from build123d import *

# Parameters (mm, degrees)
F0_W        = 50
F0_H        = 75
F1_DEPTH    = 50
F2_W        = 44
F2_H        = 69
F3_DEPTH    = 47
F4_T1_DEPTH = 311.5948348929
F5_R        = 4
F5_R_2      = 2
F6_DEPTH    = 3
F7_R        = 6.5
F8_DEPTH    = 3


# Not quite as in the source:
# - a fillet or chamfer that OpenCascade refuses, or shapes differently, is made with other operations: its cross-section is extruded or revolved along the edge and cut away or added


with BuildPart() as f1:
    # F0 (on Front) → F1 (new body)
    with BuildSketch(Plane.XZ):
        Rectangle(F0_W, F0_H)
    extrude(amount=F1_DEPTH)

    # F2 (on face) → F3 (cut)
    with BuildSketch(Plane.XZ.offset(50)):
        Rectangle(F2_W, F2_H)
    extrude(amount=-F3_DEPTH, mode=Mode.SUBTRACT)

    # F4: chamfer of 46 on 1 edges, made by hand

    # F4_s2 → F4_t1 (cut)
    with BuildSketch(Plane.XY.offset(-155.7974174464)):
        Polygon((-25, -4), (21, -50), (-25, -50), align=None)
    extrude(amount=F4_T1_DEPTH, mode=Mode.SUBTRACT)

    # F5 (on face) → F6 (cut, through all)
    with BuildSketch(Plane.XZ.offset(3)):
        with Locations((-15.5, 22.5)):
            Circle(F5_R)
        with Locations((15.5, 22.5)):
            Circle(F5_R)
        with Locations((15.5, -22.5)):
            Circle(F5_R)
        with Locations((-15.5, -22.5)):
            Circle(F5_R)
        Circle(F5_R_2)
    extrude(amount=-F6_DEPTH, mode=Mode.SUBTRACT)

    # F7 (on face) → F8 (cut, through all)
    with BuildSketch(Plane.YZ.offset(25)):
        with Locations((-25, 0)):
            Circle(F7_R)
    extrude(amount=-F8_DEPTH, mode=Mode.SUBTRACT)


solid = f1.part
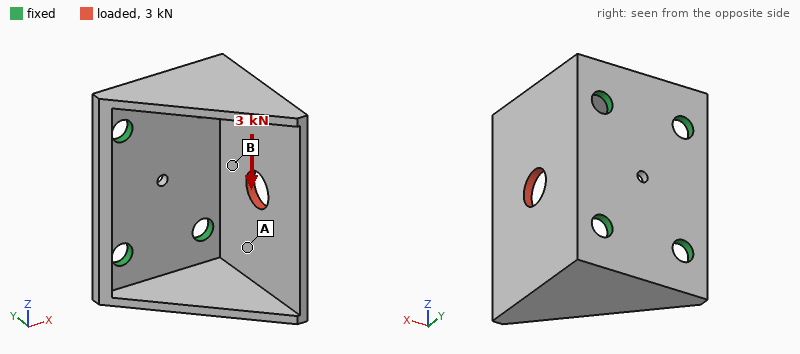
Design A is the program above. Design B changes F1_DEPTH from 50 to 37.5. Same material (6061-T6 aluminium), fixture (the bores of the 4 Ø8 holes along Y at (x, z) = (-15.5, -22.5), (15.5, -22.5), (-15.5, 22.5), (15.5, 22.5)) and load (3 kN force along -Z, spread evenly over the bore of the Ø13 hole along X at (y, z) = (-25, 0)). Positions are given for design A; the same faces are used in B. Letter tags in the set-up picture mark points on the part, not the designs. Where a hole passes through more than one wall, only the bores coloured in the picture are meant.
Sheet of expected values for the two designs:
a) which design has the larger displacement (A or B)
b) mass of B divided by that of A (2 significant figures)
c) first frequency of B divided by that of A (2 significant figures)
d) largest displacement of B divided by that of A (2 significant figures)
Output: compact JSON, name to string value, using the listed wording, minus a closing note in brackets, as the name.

{"which design has the larger displacement": "A", "mass of B divided by that of A": "0.88", "first frequency of B divided by that of A": "1.4", "largest displacement of B divided by that of A": "0.87"}
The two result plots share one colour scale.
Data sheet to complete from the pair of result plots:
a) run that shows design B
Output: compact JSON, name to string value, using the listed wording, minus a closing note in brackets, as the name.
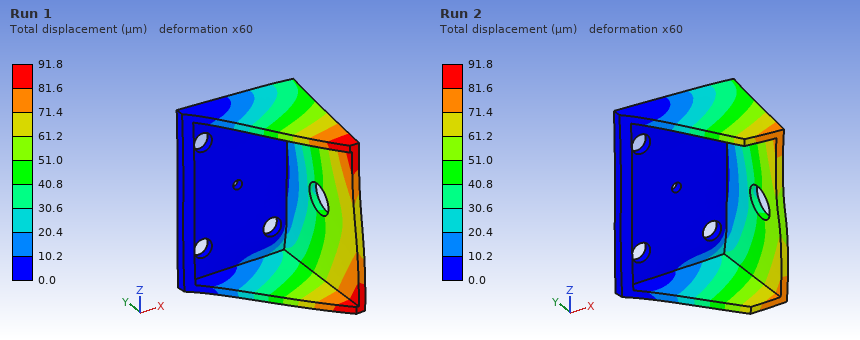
{"run that shows design B": "Run 2"}
